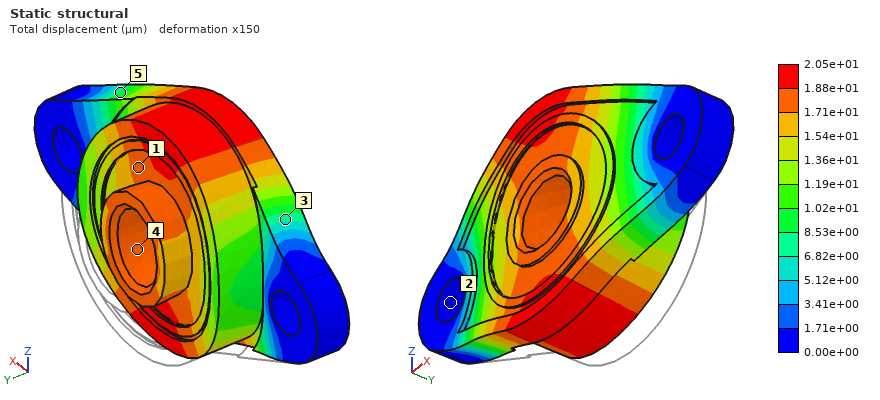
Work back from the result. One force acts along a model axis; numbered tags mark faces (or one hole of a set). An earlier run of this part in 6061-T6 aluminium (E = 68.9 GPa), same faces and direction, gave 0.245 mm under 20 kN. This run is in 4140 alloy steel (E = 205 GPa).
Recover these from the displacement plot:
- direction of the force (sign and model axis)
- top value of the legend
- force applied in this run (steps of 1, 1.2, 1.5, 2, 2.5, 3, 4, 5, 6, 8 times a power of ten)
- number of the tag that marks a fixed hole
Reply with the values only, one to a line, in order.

-Y
2.05e+01 µm
5 kN
2
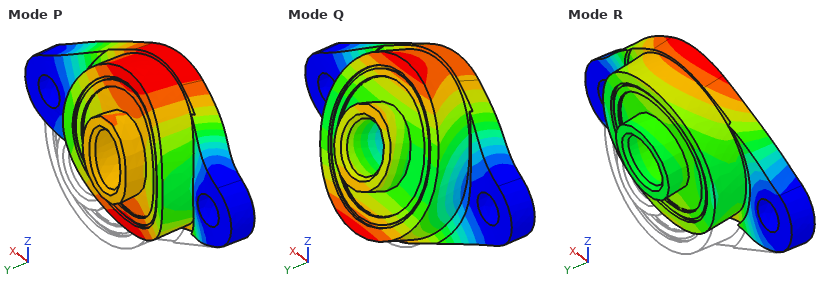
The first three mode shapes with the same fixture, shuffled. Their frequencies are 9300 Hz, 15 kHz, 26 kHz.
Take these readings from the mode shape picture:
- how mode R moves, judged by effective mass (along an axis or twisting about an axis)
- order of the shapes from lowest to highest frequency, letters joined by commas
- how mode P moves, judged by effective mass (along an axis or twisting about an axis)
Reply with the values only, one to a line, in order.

along Z
Q, P, R
along Y
